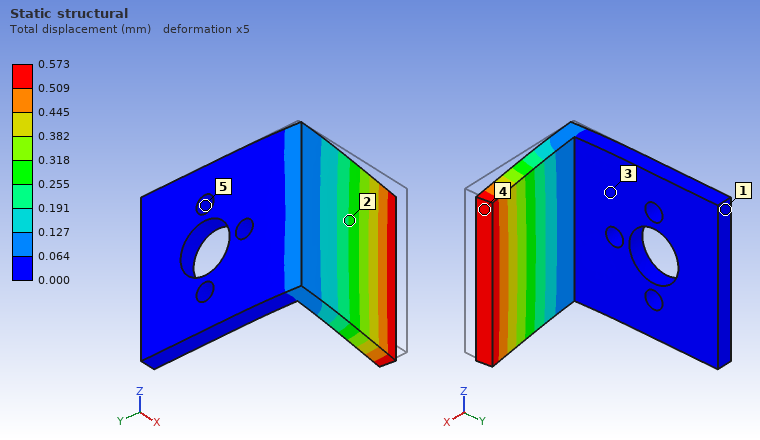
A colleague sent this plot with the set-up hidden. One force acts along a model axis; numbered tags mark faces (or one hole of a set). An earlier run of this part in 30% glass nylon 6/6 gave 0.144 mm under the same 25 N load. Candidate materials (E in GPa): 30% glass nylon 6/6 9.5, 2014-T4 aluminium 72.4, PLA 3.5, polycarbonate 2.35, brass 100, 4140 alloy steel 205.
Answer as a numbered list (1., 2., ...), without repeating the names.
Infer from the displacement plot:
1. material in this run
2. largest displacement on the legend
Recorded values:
1. polycarbonate
2. 0.573 mm
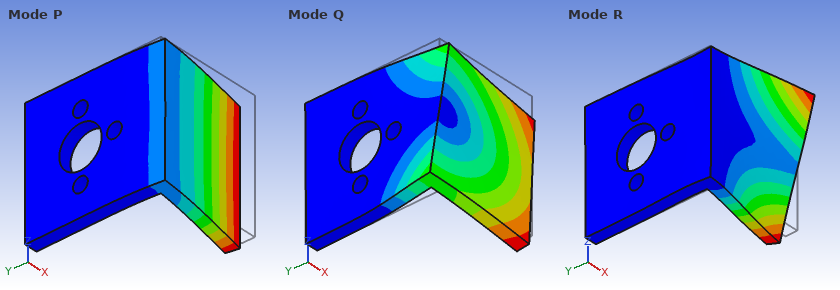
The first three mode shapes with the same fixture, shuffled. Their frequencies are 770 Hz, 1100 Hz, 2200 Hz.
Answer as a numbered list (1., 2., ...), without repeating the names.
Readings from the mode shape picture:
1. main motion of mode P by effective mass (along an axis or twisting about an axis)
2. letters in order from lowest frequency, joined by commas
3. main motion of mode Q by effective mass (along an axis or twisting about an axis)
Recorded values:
1. along Y
2. P, Q, R
3. along Z
